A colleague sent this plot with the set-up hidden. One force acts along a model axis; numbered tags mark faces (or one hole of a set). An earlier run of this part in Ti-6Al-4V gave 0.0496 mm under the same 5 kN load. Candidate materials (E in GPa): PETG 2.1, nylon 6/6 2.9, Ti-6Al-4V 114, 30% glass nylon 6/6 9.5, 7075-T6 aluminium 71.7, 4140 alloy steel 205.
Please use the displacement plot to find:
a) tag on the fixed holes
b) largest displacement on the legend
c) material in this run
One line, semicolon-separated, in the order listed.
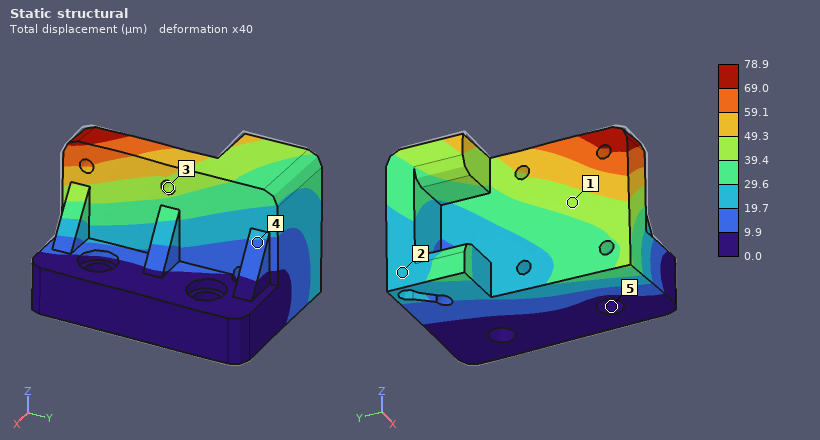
5; 78.9 µm; 7075-T6 aluminium
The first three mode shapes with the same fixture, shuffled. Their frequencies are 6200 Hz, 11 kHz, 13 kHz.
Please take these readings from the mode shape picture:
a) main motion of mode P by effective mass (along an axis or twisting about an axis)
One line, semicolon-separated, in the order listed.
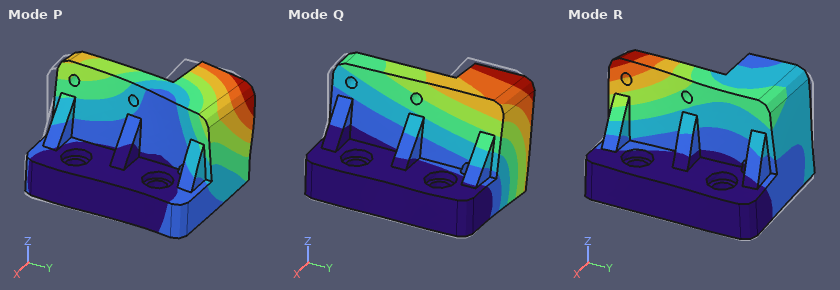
along Y
